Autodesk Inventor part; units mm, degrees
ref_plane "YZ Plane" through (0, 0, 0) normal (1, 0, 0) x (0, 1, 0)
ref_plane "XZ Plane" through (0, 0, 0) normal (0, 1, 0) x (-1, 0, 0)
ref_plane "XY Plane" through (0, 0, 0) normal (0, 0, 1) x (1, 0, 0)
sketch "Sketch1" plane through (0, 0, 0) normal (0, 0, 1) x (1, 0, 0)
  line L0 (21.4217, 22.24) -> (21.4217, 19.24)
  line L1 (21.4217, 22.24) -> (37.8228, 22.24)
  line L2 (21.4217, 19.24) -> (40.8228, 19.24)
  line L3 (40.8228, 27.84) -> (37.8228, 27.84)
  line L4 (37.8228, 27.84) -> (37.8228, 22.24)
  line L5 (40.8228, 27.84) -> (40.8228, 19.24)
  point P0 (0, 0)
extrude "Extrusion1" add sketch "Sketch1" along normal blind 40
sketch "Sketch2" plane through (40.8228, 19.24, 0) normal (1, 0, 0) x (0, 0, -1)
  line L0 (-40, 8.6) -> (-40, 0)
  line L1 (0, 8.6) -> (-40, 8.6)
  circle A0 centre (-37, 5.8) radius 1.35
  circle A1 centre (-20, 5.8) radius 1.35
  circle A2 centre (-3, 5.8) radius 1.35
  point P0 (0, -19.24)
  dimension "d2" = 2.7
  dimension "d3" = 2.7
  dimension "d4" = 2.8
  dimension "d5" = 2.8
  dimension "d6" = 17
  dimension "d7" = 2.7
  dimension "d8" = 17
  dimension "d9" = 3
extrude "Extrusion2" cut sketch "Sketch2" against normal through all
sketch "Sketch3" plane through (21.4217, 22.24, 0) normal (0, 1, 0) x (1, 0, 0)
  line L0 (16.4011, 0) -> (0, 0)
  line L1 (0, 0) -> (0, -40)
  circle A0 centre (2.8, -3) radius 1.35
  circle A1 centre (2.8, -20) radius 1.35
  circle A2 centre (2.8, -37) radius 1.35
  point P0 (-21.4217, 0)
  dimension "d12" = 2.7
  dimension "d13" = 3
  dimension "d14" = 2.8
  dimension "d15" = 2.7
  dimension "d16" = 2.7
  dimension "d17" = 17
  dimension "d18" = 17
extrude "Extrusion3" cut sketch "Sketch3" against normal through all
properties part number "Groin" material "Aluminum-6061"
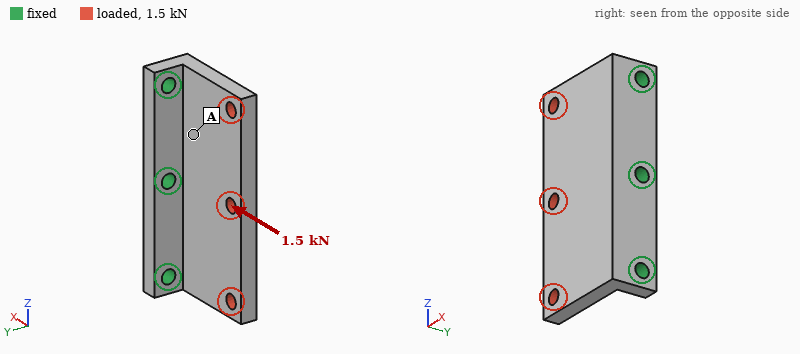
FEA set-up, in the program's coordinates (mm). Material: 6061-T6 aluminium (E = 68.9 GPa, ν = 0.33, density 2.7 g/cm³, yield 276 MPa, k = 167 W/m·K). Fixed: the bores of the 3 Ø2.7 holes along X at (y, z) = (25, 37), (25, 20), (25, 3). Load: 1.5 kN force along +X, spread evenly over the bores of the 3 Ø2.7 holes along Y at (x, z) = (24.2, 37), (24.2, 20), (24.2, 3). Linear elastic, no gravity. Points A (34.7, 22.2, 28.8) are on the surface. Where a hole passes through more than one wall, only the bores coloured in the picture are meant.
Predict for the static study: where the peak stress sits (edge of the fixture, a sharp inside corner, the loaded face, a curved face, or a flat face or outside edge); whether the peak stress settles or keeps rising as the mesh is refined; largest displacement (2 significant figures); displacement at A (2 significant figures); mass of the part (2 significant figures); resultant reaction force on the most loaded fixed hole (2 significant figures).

edge of the fixture
keeps rising
54 µm
14 µm
7.8 g
520 N
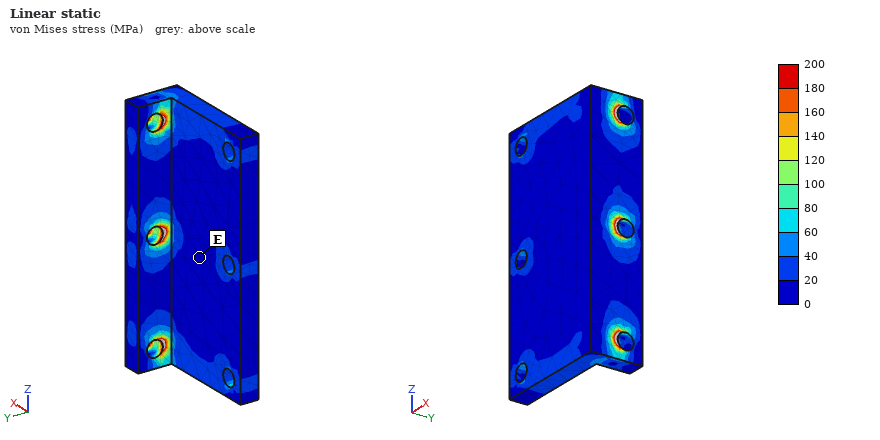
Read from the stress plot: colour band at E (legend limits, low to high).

0 to 20 MPa
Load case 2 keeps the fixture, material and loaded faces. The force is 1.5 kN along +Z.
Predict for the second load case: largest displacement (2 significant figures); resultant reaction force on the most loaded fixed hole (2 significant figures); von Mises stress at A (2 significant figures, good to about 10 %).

44 µm
790 N
41 MPa
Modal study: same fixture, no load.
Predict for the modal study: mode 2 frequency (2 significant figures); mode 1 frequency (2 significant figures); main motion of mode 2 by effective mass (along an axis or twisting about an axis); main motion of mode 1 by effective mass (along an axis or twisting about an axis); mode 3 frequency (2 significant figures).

9300 Hz
5700 Hz
twisting about X
along Y
18 kHz
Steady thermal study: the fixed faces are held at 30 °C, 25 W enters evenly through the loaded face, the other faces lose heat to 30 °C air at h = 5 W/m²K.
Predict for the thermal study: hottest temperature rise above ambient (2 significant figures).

32 K
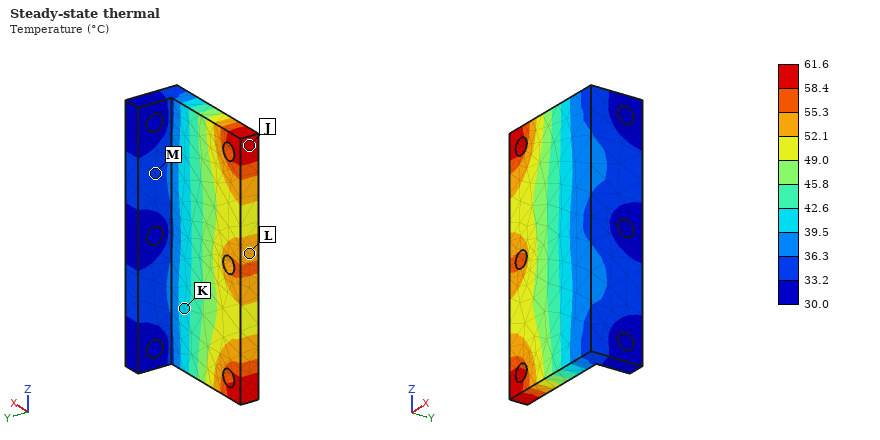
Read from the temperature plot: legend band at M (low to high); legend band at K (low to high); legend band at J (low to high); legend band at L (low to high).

33.2 to 36.3 °C
39.5 to 42.6 °C
58.4 to 61.6 °C
52.1 to 55.3 °C
